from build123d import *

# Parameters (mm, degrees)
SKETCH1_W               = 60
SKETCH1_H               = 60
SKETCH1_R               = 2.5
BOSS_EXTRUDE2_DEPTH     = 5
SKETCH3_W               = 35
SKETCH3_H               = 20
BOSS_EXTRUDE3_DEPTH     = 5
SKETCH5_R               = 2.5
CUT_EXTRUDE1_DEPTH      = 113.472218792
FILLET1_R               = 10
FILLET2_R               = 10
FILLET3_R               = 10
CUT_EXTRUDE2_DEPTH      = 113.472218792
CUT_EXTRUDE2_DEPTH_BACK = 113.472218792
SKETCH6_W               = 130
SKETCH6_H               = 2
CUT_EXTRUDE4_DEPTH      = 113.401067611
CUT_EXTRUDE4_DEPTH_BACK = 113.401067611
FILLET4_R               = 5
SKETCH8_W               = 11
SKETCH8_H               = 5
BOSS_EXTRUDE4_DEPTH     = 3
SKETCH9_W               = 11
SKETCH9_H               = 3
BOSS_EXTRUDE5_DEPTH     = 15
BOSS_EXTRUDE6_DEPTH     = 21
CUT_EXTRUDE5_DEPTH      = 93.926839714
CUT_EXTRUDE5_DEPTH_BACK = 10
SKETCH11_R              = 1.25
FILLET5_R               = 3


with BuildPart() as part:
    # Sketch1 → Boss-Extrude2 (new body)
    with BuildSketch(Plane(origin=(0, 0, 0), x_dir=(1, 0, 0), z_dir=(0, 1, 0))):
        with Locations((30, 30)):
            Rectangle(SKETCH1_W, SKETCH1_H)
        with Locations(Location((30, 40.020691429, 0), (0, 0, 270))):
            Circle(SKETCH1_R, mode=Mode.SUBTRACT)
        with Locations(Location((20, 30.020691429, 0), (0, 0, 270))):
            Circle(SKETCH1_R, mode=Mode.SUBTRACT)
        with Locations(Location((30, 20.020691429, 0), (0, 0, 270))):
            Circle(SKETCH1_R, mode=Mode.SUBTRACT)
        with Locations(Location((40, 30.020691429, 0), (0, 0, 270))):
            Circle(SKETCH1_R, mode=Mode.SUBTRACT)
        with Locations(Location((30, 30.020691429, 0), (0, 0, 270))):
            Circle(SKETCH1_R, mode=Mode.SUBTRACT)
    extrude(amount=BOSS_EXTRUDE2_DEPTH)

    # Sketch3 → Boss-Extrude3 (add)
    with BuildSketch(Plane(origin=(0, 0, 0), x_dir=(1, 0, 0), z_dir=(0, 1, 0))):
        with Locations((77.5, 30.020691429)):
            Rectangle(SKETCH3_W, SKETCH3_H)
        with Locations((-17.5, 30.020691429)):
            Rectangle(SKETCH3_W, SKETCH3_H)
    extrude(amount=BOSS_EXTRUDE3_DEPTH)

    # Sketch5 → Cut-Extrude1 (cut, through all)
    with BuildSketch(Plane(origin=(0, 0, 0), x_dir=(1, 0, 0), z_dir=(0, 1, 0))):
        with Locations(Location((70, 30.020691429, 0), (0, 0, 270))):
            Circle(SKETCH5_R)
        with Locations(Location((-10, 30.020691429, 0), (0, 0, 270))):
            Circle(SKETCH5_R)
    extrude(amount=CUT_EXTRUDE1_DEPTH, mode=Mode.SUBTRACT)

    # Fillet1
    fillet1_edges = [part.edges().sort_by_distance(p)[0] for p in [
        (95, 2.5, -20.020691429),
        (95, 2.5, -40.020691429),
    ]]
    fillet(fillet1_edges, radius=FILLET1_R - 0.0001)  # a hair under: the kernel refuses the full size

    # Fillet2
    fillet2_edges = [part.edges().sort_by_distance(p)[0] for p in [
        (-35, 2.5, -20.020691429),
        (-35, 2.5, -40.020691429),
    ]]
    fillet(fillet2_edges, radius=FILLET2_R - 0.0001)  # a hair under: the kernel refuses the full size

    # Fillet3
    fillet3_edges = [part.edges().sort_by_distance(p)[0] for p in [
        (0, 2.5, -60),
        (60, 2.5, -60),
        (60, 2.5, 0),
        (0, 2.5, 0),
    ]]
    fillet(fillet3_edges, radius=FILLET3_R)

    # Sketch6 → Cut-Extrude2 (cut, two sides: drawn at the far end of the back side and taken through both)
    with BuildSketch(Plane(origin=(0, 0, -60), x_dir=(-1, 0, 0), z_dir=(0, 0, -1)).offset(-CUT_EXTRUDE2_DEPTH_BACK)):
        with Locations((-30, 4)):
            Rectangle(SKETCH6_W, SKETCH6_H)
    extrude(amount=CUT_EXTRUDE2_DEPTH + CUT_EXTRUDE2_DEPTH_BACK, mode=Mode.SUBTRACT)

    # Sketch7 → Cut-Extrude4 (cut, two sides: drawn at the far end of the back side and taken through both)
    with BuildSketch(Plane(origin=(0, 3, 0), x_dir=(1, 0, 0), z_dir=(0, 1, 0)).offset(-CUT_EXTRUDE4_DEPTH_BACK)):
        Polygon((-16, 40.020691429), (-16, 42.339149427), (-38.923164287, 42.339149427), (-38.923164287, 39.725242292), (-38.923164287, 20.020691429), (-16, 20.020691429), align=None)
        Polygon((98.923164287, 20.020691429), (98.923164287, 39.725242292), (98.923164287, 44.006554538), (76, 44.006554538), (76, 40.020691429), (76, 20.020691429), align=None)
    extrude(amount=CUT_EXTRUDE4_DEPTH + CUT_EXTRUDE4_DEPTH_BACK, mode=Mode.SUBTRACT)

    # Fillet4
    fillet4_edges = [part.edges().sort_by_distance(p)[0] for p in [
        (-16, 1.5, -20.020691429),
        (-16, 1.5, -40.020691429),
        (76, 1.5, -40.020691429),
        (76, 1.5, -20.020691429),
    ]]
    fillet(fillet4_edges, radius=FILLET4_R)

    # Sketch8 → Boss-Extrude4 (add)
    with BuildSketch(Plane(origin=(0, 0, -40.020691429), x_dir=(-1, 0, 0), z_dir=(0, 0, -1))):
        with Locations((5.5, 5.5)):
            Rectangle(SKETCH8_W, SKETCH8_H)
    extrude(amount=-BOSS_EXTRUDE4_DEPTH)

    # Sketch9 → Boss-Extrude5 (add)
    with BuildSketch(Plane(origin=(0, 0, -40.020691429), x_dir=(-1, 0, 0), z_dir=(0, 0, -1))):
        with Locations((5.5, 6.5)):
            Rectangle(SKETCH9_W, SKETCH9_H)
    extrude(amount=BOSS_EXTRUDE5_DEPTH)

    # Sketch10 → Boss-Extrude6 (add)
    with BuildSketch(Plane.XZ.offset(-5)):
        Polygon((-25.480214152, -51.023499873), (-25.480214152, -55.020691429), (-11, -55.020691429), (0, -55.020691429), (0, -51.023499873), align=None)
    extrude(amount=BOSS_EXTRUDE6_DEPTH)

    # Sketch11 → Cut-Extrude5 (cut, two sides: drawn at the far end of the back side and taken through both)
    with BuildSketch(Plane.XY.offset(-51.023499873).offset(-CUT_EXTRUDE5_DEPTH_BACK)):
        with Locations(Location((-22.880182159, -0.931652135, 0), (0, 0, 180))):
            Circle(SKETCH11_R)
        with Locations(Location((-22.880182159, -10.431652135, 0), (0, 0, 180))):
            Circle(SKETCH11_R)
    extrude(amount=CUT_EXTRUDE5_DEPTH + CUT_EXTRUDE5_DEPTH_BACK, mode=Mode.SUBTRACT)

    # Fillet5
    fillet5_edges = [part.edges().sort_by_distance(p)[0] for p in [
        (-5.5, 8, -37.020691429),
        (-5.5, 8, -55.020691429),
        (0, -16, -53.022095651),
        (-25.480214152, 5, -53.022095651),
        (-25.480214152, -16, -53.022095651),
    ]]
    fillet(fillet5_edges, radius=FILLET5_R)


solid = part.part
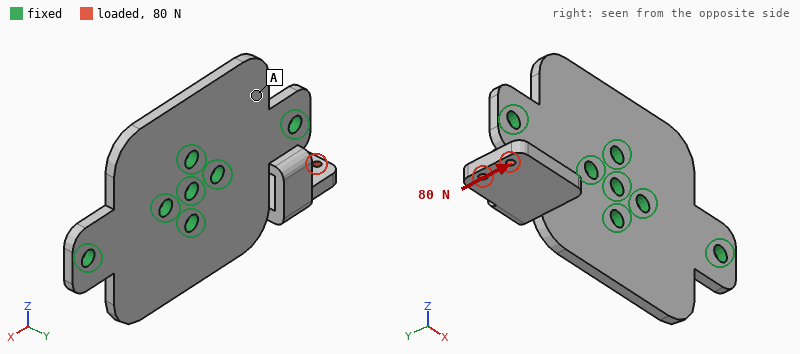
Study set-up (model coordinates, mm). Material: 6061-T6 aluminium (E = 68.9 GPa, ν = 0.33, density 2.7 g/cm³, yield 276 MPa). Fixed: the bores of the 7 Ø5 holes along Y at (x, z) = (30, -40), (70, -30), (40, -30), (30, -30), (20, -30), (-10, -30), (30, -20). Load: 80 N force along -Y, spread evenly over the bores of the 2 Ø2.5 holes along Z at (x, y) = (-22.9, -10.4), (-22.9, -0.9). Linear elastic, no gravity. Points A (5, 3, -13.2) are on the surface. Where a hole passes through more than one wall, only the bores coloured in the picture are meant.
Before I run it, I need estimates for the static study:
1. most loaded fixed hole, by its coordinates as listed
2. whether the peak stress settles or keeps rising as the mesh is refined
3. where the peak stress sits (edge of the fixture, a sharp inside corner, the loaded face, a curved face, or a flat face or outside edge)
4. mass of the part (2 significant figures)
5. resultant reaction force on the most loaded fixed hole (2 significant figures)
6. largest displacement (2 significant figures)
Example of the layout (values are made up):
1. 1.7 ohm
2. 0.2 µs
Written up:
1. (-10, -30)
2. keeps rising
3. edge of the fixture
4. 40 g
5. 100 N
6. 0.42 mm
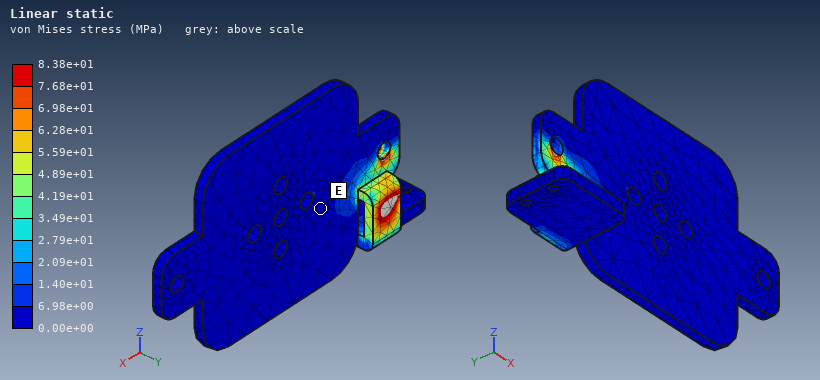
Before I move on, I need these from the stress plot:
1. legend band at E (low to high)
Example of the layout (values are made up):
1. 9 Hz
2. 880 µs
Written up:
1. 0.00e+00 to 6.98e+00 MPa
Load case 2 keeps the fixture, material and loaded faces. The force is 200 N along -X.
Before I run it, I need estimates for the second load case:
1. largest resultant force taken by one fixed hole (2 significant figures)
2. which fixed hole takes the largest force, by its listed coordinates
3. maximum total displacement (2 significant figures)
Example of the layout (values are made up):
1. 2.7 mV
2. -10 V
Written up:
1. 210 N
2. (-10, -30)
3. 0.55 mm
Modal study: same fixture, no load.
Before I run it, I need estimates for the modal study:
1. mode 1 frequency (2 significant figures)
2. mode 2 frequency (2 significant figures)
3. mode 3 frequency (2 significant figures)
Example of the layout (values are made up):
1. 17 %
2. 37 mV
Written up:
1. 1100 Hz
2. 1500 Hz
3. 3200 Hz
